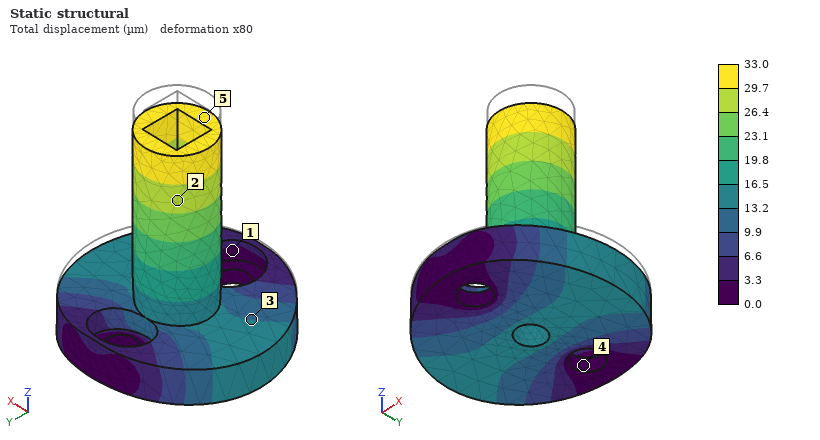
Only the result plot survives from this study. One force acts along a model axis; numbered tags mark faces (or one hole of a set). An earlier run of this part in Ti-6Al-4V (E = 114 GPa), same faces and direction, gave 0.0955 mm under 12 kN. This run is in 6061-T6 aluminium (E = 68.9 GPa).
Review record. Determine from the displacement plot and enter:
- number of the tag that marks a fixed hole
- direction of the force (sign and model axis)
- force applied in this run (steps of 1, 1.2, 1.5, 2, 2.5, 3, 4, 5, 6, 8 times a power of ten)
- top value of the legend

4
-Z
2.5 kN
33.0 µm
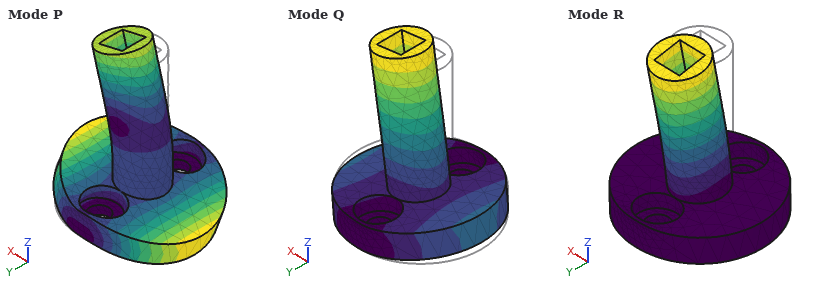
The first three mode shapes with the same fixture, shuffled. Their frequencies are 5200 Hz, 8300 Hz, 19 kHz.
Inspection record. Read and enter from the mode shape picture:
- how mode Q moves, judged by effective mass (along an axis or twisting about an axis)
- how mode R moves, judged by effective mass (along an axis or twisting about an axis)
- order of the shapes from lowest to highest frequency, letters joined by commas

along X
along Y
Q, R, P
